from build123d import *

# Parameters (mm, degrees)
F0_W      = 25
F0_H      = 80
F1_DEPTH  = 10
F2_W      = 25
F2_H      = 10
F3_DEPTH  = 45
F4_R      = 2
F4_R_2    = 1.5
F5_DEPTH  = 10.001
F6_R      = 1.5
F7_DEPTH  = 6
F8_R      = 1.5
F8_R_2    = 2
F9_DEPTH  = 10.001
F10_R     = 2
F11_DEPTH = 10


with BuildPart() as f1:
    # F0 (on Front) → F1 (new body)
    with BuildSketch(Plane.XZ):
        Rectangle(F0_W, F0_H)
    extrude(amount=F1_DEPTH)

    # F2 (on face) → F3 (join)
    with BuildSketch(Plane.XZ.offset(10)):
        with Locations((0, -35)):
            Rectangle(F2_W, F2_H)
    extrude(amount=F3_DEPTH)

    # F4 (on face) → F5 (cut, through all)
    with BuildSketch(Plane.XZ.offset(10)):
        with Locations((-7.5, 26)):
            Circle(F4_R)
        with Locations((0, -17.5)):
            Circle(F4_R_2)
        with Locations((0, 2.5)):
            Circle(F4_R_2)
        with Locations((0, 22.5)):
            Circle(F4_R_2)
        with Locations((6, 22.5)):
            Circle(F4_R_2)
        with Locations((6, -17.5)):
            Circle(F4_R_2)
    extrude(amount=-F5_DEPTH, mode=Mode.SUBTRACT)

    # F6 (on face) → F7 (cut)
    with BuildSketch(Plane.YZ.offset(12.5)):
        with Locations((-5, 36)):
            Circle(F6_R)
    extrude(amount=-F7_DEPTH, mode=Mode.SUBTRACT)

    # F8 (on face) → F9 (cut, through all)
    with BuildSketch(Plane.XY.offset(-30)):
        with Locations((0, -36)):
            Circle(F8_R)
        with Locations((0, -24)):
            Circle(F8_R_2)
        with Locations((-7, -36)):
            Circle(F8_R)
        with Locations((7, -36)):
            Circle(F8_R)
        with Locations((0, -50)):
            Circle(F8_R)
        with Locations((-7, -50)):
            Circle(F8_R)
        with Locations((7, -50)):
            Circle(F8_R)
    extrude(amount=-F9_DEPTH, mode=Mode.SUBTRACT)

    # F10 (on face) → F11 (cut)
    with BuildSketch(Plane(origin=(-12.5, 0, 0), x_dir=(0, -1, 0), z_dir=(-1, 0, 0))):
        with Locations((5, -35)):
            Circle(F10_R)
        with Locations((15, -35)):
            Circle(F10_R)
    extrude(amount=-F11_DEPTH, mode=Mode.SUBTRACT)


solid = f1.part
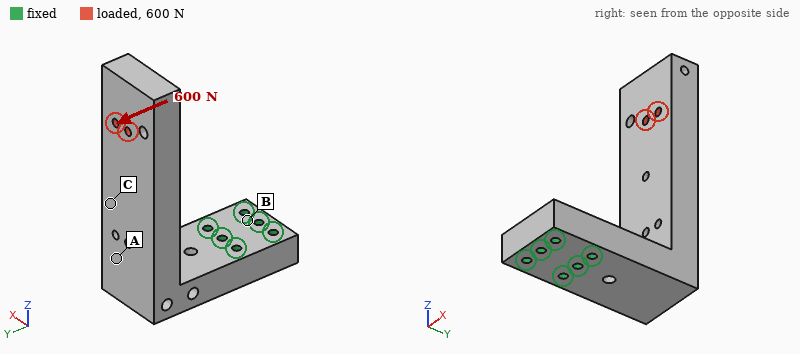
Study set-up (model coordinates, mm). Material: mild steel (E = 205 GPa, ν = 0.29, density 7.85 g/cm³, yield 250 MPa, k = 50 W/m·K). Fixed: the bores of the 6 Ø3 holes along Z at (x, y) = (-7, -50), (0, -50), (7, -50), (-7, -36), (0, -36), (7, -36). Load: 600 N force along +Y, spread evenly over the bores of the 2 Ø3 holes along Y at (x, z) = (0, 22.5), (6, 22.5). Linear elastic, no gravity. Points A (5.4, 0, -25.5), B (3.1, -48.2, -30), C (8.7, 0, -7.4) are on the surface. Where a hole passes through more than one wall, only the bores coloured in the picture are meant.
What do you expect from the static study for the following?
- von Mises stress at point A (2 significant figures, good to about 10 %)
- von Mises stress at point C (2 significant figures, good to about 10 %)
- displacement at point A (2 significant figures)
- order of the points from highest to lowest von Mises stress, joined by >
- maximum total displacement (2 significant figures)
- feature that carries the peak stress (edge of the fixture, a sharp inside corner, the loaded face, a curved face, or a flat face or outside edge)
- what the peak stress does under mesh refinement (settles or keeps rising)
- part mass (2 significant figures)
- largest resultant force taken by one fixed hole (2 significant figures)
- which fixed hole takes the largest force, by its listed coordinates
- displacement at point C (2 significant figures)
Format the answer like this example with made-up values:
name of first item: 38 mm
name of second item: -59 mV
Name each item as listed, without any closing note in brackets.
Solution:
von Mises stress at point A: 68 MPa
von Mises stress at point C: 44 MPa
displacement at point A: 0.062 mm
order of the points from highest to lowest von Mises stress, joined by >: A > C > B
maximum total displacement: 0.33 mm
feature that carries the peak stress: a sharp inside corner
what the peak stress does under mesh refinement: keeps rising
part mass: 230 g
largest resultant force taken by one fixed hole: 370 N
which fixed hole takes the largest force, by its listed coordinates: (0, -36)
displacement at point C: 0.11 mm
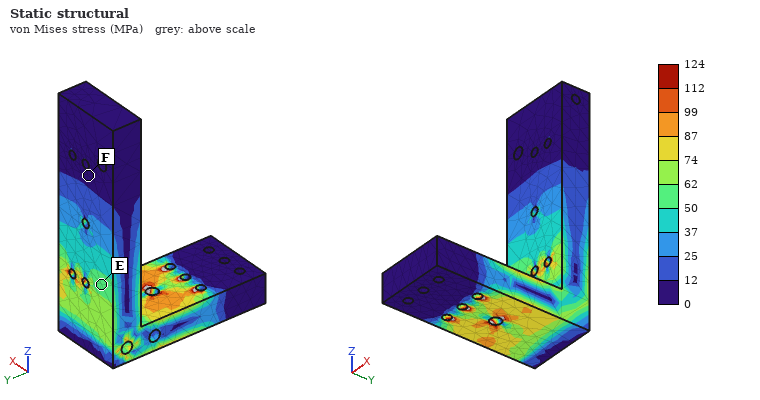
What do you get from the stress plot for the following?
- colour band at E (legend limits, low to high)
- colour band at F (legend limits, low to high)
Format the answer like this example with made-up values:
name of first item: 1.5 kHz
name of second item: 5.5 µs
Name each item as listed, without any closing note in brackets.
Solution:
colour band at E: 50 to 62 MPa
colour band at F: 0 to 12 MPa
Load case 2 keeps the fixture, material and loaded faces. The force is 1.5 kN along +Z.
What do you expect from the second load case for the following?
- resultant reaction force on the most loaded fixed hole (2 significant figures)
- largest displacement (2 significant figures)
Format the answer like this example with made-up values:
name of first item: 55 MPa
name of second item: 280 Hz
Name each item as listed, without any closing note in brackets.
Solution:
resultant reaction force on the most loaded fixed hole: 760 N
largest displacement: 0.14 mm
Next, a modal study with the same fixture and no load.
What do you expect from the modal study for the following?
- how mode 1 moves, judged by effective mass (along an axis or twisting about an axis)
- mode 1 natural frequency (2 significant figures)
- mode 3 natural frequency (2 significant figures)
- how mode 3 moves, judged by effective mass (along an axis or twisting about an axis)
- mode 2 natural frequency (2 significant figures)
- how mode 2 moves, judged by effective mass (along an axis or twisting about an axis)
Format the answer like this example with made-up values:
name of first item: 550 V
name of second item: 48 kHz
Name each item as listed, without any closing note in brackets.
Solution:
how mode 1 moves, judged by effective mass: along Y
mode 1 natural frequency: 890 Hz
mode 3 natural frequency: 3400 Hz
how mode 3 moves, judged by effective mass: along Z
mode 2 natural frequency: 1200 Hz
how mode 2 moves, judged by effective mass: along X
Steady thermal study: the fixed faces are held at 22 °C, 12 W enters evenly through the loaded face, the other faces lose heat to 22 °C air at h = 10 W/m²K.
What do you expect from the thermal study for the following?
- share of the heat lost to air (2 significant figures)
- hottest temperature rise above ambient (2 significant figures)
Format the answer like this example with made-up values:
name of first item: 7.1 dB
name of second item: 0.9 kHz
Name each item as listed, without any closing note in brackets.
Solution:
share of the heat lost to air: 27 %
hottest temperature rise above ambient: 71 K
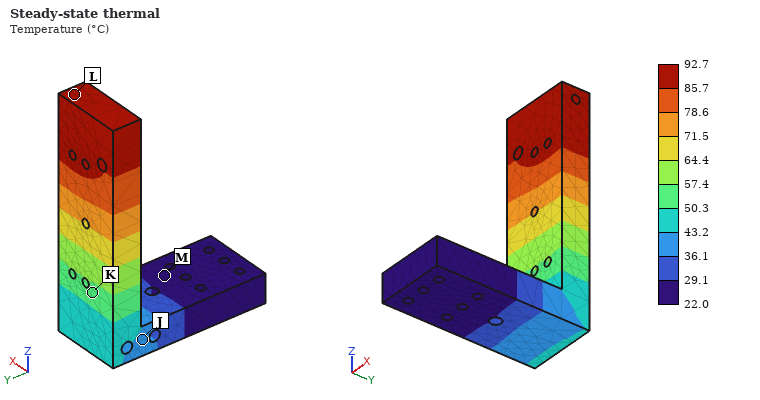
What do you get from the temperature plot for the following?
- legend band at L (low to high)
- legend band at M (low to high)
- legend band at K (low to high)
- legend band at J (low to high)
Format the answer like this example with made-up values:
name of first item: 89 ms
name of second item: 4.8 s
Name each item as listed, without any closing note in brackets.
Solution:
legend band at L: 85.7 to 92.7 °C
legend band at M: 22.0 to 29.1 °C
legend band at K: 50.3 to 57.4 °C
legend band at J: 36.1 to 43.2 °C
